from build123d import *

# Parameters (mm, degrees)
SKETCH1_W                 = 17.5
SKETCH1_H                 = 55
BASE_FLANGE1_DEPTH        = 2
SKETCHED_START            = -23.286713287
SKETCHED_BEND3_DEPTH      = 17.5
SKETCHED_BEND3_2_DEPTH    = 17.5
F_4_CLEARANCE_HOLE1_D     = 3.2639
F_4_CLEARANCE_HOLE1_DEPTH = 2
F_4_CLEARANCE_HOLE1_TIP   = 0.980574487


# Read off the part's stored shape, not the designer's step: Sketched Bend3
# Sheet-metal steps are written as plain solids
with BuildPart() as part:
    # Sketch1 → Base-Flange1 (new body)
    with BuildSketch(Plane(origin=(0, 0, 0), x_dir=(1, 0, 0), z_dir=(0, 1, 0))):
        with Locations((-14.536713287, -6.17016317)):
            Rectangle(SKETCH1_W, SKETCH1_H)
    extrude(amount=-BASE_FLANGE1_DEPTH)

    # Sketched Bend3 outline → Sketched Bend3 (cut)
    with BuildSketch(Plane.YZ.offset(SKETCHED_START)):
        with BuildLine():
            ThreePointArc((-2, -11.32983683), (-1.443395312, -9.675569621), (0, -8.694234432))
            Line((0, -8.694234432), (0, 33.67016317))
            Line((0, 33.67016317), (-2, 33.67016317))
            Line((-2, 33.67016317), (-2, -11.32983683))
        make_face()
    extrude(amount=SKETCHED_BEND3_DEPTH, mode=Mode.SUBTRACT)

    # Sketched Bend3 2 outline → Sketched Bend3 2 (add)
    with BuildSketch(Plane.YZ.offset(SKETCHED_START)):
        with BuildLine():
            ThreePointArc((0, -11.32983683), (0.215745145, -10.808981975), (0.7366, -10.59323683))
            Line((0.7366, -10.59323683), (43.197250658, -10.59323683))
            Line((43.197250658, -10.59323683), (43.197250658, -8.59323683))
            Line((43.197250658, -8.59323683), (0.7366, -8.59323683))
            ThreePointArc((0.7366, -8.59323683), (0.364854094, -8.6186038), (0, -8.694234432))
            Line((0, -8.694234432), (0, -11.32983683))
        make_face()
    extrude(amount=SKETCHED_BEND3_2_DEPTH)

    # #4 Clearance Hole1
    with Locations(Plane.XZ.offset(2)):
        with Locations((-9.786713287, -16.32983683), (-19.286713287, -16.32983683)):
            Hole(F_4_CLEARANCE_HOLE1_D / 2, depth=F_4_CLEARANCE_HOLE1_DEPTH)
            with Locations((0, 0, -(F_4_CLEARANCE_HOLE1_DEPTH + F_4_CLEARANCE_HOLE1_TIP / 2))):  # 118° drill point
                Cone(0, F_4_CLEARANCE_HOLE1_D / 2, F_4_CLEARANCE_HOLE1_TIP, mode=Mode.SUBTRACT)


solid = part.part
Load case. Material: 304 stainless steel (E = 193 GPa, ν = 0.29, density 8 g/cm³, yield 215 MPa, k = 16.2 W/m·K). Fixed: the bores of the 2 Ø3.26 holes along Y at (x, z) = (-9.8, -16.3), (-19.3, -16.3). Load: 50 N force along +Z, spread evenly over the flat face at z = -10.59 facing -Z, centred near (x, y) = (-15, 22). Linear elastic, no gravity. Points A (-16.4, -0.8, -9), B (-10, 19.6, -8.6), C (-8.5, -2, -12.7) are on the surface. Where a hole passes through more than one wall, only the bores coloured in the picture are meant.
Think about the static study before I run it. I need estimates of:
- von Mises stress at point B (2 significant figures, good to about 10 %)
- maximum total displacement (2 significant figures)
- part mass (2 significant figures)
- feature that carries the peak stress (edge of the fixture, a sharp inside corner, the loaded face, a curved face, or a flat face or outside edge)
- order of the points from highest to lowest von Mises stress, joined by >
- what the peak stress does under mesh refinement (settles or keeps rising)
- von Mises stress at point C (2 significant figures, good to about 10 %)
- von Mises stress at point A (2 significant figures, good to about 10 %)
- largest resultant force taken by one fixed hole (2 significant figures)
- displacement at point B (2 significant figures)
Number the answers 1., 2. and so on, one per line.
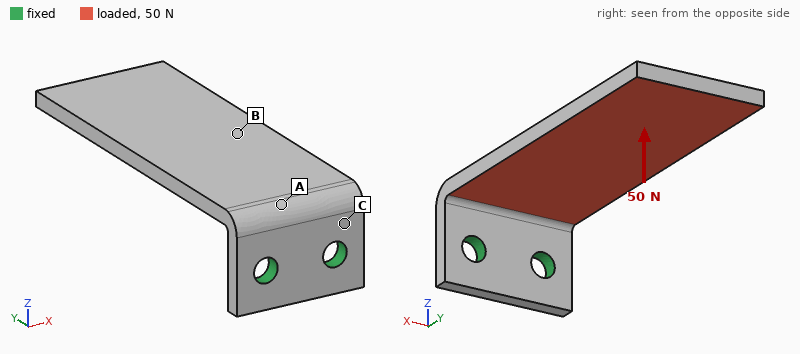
1. 28 MPa
2. 0.35 mm
3. 15 g
4. edge of the fixture
5. C > A > B
6. keeps rising
7. 91 MPa
8. 63 MPa
9. 31 N
10. 0.13 mm
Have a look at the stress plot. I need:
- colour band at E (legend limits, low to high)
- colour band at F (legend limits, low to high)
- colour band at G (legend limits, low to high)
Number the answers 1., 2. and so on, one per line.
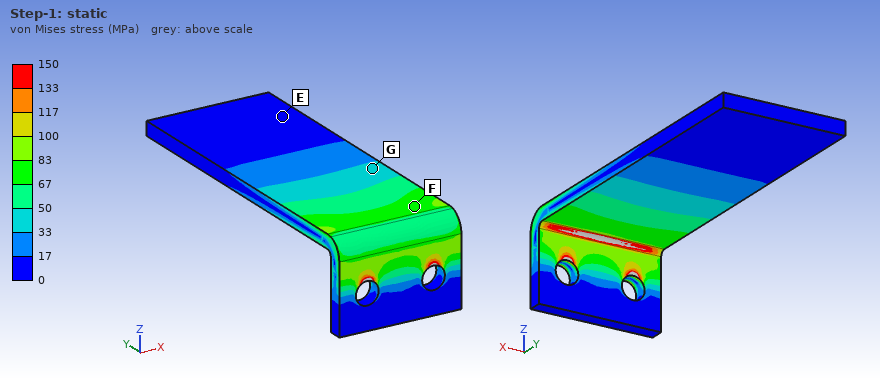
1. 0 to 17 MPa
2. 67 to 83 MPa
3. 33 to 50 MPa
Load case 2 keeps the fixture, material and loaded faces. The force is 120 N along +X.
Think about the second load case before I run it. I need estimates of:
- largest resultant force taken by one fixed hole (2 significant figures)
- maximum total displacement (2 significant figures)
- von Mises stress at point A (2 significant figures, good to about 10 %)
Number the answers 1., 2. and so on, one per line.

1. 250 N
2. 78 µm
3. 55 MPa
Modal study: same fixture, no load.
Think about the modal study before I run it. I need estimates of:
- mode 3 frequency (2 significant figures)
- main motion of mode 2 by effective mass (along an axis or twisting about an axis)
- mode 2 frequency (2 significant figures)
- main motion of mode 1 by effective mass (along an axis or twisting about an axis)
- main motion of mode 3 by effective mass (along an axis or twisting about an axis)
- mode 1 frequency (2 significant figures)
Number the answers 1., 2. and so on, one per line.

1. 4200 Hz
2. along X
3. 2300 Hz
4. along Z
5. twisting about Y
6. 680 Hz
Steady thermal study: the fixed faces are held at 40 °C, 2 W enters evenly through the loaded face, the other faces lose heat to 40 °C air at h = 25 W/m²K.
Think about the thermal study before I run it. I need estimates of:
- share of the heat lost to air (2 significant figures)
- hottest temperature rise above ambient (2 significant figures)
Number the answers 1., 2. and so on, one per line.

1. 47 %
2. 48 K
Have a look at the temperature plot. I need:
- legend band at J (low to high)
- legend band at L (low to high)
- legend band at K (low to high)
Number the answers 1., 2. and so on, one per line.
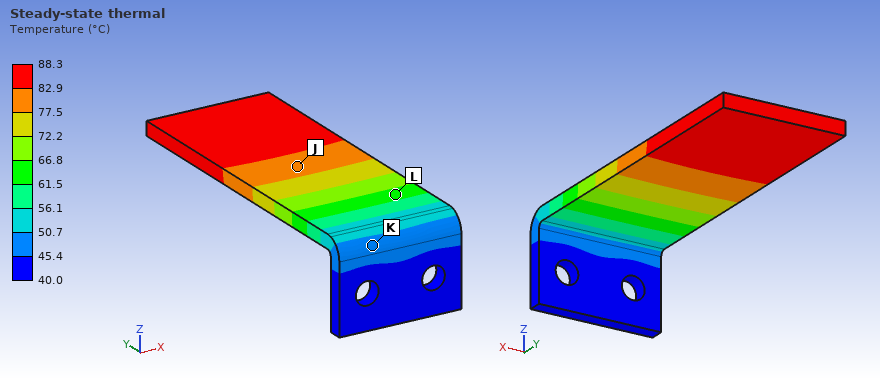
1. 77.5 to 82.9 °C
2. 61.5 to 66.8 °C
3. 45.4 to 50.7 °C
